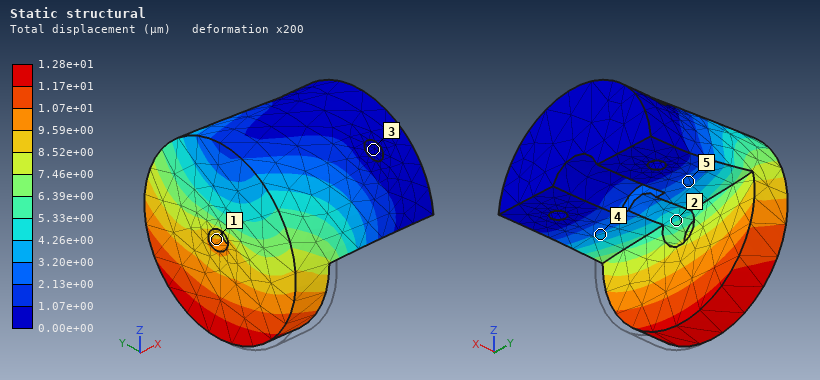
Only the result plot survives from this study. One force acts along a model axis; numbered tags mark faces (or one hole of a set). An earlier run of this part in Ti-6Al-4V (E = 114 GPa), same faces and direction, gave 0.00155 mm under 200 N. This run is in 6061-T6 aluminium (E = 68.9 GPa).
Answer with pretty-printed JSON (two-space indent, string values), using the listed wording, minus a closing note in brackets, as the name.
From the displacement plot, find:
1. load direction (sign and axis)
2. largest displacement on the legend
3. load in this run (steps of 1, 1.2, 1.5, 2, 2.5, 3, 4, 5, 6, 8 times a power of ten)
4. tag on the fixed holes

{
  "load direction": "+Y",
  "largest displacement on the legend": "1.28e+01 µm",
  "load in this run": "1 kN",
  "tag on the fixed holes": "3"
}
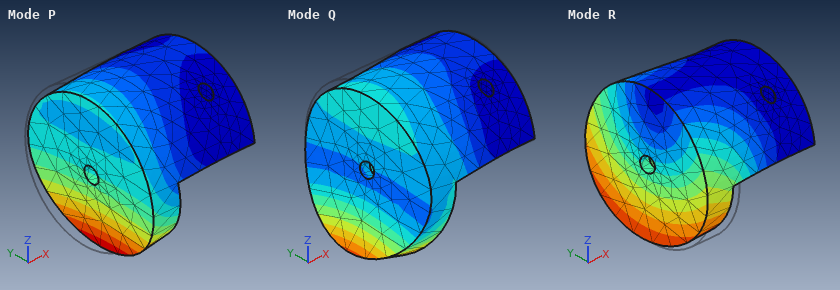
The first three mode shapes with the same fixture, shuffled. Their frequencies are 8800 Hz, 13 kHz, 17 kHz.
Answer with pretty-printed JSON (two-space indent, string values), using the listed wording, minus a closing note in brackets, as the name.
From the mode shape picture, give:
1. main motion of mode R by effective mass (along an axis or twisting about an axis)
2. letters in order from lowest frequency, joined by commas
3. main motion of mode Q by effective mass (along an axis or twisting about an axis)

{
  "main motion of mode R by effective mass": "along Y",
  "letters in order from lowest frequency, joined by commas": "P, R, Q",
  "main motion of mode Q by effective mass": "along Z"
}
